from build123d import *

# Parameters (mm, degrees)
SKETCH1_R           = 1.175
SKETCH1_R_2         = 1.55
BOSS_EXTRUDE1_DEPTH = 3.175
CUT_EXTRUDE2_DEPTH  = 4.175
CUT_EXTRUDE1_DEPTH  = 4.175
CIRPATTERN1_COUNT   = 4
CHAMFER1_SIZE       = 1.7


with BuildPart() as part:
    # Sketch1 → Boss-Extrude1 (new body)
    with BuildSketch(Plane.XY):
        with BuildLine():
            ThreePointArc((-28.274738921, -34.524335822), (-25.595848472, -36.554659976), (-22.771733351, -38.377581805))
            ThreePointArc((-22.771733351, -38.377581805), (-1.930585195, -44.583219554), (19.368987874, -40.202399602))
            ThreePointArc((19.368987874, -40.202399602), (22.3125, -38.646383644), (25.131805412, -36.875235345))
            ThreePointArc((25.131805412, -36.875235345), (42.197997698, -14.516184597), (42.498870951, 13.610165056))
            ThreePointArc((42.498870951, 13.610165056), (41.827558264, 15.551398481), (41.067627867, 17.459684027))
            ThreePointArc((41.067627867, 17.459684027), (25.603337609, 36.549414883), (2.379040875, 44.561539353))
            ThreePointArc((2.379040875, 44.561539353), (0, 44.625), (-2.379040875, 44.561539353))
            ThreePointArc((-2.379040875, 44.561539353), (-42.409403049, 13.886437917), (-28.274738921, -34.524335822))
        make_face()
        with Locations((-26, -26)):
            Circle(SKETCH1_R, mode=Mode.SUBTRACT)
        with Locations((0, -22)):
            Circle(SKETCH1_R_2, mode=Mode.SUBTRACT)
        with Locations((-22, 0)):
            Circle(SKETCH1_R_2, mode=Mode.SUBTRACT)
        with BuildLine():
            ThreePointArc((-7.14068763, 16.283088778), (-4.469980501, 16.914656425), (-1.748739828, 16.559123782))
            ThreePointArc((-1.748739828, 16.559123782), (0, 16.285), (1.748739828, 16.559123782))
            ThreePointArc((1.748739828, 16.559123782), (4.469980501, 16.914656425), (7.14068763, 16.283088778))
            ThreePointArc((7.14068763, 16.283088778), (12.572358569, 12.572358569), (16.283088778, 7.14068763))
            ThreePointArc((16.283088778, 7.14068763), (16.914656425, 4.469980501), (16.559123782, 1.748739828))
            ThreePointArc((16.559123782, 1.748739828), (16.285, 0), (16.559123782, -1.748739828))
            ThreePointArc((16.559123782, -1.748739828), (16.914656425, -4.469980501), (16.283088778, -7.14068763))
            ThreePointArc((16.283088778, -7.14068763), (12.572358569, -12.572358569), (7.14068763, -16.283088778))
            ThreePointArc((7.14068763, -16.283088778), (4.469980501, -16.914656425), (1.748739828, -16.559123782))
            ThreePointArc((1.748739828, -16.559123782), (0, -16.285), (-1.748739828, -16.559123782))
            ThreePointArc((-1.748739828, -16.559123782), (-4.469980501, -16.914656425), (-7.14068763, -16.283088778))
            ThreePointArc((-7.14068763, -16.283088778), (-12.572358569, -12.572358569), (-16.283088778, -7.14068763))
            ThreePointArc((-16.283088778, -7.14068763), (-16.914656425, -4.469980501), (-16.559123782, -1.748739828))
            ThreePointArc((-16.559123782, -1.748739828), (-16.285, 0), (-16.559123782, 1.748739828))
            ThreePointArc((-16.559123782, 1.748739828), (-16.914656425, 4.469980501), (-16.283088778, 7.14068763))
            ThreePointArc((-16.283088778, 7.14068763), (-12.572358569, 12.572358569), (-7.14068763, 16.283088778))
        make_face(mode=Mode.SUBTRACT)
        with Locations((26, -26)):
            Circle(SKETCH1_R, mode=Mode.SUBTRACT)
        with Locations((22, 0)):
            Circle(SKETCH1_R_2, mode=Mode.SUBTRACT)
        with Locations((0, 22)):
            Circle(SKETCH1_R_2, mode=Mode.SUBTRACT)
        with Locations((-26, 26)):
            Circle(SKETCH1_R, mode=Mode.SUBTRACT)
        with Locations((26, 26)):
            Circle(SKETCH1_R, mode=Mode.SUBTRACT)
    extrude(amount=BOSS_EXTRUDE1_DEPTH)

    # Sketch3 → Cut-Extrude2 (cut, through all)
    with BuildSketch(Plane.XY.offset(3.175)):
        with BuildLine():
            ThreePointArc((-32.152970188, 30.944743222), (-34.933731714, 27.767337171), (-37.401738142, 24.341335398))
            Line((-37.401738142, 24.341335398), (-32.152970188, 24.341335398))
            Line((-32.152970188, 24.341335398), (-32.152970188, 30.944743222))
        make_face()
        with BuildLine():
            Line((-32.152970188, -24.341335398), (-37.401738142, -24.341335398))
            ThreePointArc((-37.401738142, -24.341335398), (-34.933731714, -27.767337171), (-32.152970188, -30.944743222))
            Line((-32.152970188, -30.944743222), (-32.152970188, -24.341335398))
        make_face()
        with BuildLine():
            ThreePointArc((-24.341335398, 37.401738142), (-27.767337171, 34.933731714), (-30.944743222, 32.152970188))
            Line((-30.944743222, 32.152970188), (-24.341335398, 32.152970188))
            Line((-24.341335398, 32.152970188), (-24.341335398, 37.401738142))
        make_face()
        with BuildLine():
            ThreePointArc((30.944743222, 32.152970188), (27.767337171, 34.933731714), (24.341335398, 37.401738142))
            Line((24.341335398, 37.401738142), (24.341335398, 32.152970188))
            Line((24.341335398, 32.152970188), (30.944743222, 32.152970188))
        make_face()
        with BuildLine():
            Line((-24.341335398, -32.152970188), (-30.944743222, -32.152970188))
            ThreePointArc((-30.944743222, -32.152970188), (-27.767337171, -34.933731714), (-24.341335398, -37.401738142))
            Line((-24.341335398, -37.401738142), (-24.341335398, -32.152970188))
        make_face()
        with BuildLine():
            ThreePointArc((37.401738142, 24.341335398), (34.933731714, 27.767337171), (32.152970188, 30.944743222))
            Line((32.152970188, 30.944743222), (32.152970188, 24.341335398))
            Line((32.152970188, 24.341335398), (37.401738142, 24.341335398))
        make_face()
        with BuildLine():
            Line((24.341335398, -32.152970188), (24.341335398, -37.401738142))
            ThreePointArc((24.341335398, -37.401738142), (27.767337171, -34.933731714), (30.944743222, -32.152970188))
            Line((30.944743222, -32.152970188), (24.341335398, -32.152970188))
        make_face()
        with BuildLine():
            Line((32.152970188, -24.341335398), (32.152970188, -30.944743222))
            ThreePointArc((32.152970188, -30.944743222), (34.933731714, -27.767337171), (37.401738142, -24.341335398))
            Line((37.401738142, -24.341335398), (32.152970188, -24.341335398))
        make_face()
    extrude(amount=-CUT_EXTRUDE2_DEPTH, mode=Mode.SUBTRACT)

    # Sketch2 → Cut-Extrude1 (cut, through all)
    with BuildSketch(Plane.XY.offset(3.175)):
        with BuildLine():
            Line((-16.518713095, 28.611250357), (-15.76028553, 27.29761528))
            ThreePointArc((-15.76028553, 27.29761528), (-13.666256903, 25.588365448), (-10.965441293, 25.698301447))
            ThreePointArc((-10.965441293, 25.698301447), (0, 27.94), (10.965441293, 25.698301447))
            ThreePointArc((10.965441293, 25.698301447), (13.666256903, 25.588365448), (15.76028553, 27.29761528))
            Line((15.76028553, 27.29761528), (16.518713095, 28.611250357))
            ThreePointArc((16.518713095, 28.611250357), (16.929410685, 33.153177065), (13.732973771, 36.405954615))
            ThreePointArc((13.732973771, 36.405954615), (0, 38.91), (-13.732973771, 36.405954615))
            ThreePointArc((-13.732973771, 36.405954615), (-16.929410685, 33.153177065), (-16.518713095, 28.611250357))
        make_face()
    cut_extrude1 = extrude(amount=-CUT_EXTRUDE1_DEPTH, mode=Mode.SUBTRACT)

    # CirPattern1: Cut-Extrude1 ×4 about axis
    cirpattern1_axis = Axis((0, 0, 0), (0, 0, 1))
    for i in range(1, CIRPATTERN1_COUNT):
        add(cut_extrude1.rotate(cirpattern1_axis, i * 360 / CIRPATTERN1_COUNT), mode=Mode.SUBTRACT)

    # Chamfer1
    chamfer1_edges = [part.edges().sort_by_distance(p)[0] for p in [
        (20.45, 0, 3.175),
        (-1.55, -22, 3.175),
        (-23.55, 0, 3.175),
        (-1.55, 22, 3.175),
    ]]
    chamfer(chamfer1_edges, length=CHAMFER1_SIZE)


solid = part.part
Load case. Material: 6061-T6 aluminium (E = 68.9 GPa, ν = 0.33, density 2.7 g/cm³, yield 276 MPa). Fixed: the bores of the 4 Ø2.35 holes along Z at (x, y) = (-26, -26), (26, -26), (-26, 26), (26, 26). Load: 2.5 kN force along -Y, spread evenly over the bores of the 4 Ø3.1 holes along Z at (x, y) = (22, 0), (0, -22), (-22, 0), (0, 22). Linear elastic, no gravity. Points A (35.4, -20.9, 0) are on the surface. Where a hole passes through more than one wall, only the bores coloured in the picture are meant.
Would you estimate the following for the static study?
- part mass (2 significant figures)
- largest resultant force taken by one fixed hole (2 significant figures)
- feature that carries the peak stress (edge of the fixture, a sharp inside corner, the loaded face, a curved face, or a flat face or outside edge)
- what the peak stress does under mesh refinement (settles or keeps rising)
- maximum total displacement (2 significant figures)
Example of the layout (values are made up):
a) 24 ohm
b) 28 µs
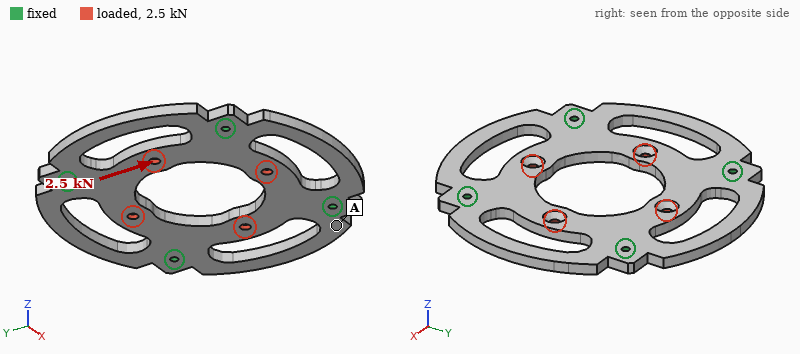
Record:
a) 31 g
b) 650 N
c) edge of the fixture
d) keeps rising
e) 25 µm
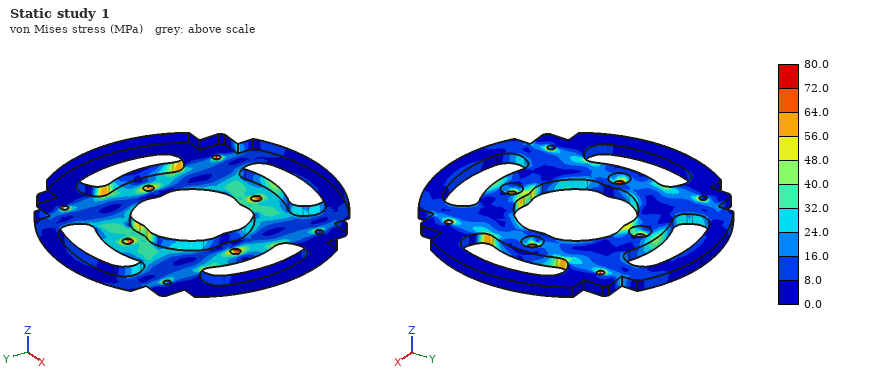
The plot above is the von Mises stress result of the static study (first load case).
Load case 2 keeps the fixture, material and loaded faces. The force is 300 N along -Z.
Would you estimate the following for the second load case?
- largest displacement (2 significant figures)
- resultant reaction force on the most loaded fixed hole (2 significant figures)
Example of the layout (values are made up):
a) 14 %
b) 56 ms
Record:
a) 44 µm
b) 77 N
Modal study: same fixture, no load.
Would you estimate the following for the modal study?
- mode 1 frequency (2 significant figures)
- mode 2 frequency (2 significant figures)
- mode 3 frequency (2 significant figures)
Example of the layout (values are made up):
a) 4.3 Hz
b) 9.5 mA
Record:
a) 4000 Hz
b) 4200 Hz
c) 4200 Hz
